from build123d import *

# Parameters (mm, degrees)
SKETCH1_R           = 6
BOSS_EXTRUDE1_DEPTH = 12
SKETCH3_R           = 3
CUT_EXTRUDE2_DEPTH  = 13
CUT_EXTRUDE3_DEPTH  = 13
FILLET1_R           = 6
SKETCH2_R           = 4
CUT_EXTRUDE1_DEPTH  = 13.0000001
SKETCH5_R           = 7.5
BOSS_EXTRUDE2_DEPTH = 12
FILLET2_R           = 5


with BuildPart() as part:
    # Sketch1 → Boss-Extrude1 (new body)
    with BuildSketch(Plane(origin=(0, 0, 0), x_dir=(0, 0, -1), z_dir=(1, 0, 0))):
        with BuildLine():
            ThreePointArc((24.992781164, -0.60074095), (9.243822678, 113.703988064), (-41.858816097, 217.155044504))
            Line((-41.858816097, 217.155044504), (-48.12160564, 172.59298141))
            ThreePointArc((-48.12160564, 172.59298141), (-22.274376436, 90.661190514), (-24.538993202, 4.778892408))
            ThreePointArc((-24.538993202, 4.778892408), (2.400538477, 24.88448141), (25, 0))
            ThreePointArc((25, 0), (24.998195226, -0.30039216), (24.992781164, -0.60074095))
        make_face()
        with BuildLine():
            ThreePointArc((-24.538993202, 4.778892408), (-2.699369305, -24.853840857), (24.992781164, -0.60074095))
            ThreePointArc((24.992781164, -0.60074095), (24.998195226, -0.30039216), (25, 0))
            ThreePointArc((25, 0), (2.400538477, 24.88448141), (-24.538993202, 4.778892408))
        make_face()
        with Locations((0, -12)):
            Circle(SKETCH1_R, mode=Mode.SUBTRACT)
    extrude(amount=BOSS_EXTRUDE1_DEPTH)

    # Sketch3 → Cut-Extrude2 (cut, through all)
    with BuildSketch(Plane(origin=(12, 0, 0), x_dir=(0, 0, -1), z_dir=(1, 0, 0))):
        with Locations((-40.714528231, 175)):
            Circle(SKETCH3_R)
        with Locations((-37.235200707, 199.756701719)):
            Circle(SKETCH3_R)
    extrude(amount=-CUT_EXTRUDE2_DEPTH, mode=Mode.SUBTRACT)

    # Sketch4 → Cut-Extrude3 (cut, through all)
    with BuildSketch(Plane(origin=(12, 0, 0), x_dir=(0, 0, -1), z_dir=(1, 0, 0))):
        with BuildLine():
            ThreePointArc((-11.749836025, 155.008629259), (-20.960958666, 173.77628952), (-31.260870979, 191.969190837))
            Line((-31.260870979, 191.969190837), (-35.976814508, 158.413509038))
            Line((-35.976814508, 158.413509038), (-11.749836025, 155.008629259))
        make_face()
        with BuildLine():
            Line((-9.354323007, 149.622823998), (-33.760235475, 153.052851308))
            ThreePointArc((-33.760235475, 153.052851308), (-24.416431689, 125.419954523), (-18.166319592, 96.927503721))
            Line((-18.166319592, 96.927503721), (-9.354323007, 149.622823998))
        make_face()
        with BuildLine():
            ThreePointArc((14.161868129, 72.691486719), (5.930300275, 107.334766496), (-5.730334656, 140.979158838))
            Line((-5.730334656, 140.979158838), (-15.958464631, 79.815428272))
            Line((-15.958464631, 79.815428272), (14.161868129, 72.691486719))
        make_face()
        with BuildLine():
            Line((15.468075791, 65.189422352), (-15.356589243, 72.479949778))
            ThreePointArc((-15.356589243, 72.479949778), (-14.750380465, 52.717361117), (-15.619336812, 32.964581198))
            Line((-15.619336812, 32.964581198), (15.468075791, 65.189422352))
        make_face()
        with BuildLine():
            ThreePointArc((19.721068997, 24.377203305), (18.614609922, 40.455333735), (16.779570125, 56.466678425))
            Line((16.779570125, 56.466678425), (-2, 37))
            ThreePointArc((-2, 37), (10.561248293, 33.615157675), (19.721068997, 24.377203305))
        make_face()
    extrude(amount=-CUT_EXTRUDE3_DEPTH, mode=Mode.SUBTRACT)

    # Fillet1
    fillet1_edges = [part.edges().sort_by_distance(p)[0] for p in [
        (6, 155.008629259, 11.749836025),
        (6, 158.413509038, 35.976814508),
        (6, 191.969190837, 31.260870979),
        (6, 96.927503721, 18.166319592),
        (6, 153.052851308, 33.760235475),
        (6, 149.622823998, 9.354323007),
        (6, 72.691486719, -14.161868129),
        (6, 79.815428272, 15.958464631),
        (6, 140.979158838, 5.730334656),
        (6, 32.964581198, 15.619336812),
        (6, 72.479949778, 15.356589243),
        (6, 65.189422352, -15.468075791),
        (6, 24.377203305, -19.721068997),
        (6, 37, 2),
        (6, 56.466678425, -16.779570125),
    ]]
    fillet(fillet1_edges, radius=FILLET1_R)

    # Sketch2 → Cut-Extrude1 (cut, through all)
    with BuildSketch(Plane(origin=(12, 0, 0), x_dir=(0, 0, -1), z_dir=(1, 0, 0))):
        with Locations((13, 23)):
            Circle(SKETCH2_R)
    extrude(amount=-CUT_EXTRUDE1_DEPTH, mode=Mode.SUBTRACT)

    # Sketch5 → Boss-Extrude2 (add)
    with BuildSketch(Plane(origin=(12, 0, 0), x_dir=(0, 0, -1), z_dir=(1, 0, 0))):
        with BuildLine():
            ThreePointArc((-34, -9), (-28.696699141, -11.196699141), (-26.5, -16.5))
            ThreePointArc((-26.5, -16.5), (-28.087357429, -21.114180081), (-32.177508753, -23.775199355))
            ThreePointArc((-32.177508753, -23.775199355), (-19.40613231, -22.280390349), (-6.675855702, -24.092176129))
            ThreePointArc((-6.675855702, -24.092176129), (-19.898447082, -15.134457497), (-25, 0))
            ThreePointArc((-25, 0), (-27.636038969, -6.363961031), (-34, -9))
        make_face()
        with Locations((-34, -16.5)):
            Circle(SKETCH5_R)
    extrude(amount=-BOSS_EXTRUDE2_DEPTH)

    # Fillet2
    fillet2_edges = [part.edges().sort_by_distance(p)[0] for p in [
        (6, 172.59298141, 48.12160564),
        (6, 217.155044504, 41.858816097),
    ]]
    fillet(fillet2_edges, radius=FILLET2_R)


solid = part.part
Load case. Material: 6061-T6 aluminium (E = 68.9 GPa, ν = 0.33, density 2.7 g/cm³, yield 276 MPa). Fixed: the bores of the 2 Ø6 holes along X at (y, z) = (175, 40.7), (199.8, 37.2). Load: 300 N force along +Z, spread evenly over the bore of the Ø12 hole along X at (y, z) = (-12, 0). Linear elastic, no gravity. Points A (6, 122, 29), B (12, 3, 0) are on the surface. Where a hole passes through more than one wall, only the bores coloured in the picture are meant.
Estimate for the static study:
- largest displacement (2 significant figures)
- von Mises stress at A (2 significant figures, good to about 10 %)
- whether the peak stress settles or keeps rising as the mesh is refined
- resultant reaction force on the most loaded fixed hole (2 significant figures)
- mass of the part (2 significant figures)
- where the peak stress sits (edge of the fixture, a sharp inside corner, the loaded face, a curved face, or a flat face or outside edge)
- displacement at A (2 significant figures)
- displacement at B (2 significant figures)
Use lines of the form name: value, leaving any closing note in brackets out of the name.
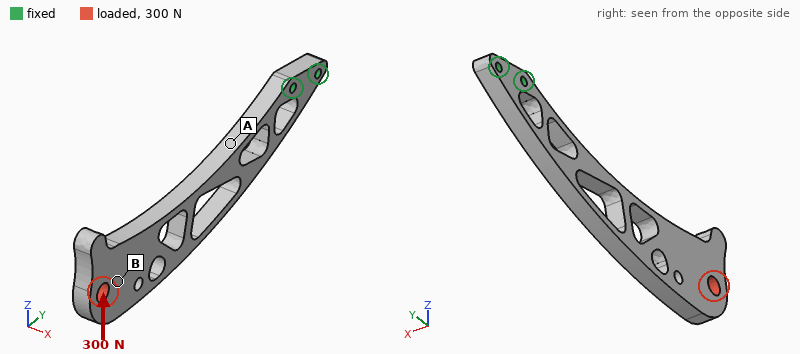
largest displacement: 0.62 mm
von Mises stress at A: 29 MPa
whether the peak stress settles or keeps rising as the mesh is refined: keeps rising
resultant reaction force on the most loaded fixed hole: 2.3 kN
mass of the part: 200 g
where the peak stress sits: edge of the fixture
displacement at A: 0.098 mm
displacement at B: 0.53 mm
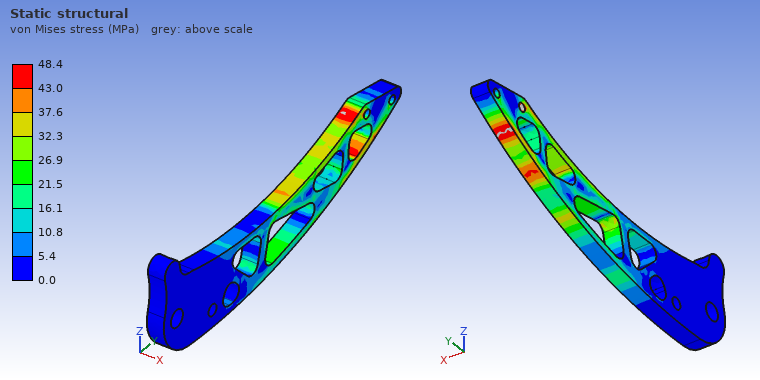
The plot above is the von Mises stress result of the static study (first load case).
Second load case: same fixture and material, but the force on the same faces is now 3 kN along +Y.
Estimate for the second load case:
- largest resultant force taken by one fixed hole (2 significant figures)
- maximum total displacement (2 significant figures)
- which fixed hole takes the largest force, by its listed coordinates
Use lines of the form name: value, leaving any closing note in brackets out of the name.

largest resultant force taken by one fixed hole: 4.7 kN
maximum total displacement: 0.88 mm
which fixed hole takes the largest force, by its listed coordinates: (199.8, 37.2)
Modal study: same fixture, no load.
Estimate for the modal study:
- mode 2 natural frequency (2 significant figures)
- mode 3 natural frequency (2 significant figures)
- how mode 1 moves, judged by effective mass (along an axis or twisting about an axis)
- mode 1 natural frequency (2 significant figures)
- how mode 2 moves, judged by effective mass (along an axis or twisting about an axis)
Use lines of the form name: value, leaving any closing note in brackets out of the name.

mode 2 natural frequency: 380 Hz
mode 3 natural frequency: 680 Hz
how mode 1 moves, judged by effective mass: along X
mode 1 natural frequency: 140 Hz
how mode 2 moves, judged by effective mass: along Z
